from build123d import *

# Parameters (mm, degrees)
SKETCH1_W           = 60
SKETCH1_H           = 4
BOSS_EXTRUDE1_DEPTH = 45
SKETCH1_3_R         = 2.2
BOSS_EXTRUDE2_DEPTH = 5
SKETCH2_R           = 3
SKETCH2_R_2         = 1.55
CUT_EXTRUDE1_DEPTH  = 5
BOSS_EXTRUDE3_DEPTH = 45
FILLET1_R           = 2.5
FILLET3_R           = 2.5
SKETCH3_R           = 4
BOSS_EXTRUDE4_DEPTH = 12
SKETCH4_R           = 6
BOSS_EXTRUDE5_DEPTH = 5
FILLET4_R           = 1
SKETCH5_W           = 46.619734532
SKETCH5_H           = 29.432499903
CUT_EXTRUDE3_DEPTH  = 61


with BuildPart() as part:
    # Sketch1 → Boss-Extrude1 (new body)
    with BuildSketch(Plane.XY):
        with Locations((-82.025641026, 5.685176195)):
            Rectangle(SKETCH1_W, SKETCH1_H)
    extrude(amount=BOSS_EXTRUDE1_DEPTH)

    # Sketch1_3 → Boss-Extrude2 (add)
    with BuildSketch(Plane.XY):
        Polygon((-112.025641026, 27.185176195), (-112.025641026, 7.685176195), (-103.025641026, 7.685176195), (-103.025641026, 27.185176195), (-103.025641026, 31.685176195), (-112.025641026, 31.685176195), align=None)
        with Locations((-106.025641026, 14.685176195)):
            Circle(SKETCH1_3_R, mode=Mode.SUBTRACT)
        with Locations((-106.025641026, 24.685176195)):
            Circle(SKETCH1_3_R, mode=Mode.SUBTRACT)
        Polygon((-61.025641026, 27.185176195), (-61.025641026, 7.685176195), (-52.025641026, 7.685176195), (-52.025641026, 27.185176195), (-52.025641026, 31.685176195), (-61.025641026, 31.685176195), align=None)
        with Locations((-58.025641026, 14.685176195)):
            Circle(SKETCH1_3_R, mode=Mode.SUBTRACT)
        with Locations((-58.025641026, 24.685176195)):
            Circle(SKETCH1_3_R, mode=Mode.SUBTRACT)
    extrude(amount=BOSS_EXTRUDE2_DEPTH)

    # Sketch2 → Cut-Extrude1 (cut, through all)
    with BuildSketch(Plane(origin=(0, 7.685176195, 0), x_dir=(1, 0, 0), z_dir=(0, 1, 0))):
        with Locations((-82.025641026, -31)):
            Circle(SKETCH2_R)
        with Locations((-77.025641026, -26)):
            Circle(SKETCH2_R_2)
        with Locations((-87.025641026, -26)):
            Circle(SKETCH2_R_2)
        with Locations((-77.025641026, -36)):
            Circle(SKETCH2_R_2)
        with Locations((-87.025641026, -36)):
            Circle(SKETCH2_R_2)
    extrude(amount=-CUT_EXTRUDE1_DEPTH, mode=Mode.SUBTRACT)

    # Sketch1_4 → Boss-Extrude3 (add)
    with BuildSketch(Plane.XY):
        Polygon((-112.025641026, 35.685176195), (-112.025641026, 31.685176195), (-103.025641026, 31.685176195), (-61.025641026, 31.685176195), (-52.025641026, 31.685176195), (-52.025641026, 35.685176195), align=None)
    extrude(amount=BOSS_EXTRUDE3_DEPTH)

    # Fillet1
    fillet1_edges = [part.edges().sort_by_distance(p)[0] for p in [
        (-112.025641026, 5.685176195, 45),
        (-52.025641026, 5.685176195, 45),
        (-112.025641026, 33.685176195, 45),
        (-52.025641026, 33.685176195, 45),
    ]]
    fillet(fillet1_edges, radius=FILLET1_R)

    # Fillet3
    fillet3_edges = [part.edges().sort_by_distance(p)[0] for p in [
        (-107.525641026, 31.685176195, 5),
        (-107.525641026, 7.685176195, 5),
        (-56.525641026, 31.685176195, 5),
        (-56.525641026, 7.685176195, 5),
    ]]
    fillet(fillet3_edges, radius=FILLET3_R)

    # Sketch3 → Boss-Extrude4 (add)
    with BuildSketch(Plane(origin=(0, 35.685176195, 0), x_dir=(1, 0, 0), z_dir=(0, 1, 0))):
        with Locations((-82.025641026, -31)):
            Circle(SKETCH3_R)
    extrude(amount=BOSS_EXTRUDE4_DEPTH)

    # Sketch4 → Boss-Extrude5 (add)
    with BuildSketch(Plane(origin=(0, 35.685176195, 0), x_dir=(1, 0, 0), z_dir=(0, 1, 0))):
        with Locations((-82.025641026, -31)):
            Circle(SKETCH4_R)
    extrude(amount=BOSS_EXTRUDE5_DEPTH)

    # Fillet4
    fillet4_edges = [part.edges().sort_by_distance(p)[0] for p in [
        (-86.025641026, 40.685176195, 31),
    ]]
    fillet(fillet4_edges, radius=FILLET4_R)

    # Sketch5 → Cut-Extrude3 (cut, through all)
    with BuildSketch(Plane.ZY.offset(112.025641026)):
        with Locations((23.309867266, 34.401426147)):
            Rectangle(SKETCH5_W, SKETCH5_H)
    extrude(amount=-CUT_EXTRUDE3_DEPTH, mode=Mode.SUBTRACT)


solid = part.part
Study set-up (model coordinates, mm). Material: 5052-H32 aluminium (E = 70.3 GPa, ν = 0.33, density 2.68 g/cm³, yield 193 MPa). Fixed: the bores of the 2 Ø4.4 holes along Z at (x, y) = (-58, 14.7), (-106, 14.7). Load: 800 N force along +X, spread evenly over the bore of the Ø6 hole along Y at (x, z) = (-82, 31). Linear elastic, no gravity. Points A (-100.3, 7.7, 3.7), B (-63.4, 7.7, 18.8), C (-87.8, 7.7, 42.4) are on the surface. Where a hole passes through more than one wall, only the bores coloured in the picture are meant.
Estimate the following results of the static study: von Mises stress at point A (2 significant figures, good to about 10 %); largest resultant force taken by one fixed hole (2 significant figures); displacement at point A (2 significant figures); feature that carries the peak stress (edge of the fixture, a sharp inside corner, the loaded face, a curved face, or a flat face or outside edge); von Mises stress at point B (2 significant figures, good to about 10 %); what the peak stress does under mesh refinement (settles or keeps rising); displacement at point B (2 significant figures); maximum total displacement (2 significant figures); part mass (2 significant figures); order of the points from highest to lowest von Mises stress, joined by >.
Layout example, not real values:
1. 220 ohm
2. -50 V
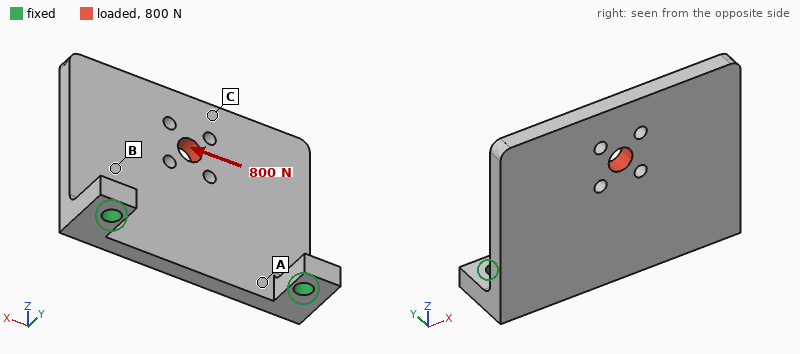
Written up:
1. 27 MPa
2. 590 N
3. 9.7 µm
4. edge of the fixture
5. 13 MPa
6. keeps rising
7. 21 µm
8. 42 µm
9. 31 g
10. A > B > C
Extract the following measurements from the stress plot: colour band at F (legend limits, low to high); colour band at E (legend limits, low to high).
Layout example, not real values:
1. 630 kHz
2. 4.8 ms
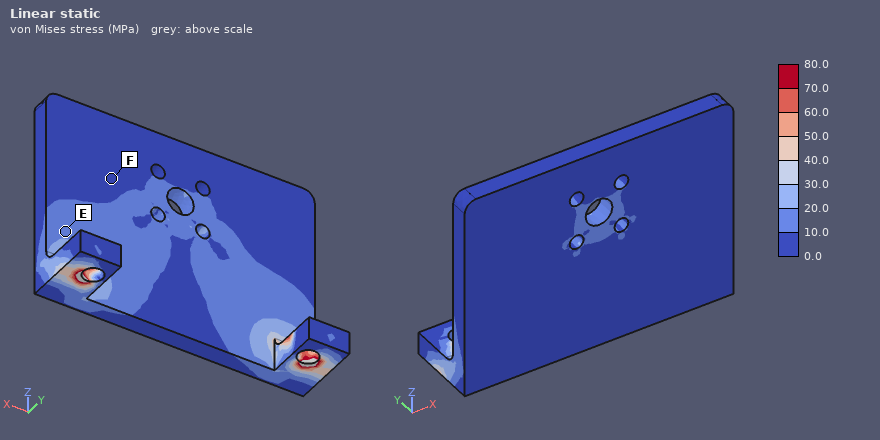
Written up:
1. 0.0 to 10.0 MPa
2. 10.0 to 20.0 MPa
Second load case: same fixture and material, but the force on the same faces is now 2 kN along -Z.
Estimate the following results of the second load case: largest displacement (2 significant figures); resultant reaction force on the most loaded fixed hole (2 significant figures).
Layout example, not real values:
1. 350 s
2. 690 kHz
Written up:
1. 0.21 mm
2. 1.0 kN
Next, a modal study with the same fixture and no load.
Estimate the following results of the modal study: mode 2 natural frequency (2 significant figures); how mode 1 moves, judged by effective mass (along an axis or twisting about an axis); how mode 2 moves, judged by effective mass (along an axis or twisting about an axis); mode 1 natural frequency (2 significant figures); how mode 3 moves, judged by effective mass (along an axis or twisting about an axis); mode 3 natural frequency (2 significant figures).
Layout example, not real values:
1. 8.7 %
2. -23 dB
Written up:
1. 3100 Hz
2. along Y
3. twisting about Z
4. 1200 Hz
5. along X
6. 6400 Hz
